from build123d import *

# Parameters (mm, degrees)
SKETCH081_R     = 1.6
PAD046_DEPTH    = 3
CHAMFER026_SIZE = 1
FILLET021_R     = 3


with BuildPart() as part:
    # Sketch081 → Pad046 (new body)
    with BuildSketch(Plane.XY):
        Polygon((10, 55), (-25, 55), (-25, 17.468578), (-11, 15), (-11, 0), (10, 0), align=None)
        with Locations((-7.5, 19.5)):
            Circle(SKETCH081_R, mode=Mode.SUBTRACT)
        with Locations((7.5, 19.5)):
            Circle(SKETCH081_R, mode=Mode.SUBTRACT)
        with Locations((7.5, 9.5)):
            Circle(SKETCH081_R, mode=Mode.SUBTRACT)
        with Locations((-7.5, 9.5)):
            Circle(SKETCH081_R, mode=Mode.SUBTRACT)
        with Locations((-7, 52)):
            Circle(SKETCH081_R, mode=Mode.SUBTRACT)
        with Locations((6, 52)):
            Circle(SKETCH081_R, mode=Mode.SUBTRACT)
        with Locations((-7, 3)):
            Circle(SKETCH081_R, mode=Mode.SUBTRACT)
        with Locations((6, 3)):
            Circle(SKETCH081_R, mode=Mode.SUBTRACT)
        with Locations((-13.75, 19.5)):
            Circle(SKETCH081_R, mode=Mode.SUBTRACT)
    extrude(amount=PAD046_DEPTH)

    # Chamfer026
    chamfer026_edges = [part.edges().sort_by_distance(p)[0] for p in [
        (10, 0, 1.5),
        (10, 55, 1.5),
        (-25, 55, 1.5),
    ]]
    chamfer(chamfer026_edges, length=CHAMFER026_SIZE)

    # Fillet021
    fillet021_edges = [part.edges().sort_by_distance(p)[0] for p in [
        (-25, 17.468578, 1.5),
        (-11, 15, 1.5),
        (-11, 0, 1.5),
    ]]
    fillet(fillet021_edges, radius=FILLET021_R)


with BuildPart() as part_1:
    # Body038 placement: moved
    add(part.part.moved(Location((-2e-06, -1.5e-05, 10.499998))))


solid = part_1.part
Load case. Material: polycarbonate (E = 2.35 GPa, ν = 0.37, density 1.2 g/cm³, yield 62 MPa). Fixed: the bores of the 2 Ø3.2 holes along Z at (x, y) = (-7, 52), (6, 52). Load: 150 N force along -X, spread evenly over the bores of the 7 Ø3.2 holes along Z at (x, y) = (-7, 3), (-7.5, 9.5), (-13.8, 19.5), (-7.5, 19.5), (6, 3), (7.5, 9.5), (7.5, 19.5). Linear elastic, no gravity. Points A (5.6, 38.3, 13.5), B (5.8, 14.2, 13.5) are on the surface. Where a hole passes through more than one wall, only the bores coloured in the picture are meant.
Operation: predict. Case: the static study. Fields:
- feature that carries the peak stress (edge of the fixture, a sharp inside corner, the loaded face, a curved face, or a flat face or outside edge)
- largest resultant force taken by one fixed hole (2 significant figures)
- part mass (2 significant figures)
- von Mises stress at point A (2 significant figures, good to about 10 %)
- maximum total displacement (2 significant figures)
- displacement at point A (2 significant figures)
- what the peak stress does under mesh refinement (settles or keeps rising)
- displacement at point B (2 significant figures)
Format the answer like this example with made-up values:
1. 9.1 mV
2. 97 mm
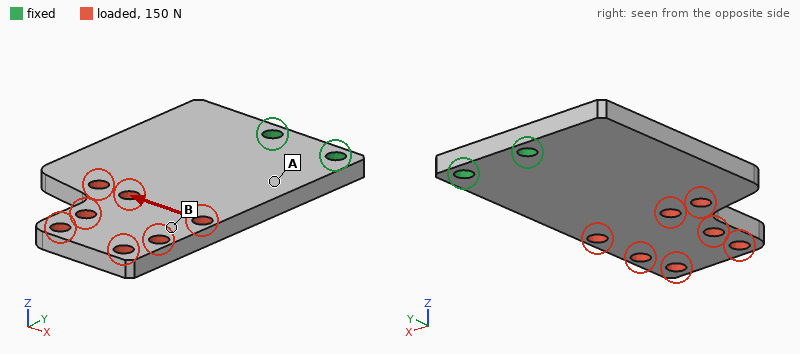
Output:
1. edge of the fixture
2. 410 N
3. 5.8 g
4. 8.4 MPa
5. 0.74 mm
6. 0.15 mm
7. keeps rising
8. 0.50 mm
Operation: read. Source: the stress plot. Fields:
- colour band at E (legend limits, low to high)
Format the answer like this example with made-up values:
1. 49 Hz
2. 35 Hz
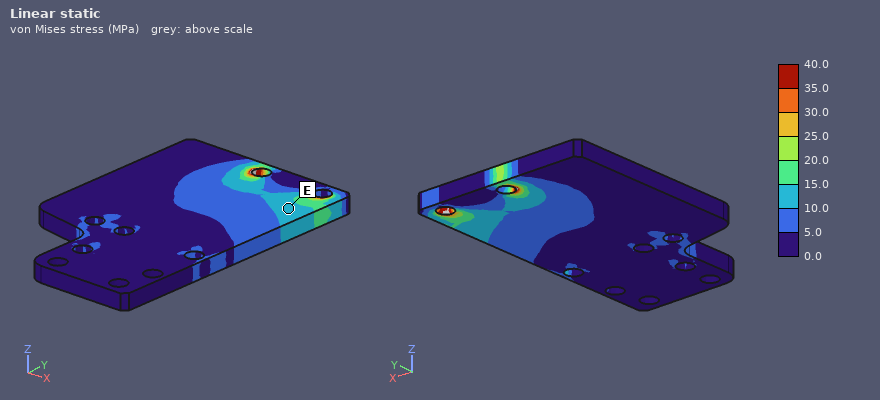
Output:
1. 10.0 to 15.0 MPa
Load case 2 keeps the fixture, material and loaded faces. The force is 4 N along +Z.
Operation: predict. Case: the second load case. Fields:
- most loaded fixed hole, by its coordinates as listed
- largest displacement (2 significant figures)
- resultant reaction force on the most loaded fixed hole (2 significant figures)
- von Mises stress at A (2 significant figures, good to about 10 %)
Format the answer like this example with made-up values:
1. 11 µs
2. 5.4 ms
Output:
1. (-7, 52)
2. 0.78 mm
3. 3.1 N
4. 2.3 MPa
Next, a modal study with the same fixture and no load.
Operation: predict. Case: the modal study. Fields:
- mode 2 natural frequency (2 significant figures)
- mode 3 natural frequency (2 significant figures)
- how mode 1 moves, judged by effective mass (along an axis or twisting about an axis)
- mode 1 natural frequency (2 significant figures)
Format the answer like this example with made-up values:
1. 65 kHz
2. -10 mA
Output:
1. 860 Hz
2. 1600 Hz
3. along Z
4. 300 Hz
